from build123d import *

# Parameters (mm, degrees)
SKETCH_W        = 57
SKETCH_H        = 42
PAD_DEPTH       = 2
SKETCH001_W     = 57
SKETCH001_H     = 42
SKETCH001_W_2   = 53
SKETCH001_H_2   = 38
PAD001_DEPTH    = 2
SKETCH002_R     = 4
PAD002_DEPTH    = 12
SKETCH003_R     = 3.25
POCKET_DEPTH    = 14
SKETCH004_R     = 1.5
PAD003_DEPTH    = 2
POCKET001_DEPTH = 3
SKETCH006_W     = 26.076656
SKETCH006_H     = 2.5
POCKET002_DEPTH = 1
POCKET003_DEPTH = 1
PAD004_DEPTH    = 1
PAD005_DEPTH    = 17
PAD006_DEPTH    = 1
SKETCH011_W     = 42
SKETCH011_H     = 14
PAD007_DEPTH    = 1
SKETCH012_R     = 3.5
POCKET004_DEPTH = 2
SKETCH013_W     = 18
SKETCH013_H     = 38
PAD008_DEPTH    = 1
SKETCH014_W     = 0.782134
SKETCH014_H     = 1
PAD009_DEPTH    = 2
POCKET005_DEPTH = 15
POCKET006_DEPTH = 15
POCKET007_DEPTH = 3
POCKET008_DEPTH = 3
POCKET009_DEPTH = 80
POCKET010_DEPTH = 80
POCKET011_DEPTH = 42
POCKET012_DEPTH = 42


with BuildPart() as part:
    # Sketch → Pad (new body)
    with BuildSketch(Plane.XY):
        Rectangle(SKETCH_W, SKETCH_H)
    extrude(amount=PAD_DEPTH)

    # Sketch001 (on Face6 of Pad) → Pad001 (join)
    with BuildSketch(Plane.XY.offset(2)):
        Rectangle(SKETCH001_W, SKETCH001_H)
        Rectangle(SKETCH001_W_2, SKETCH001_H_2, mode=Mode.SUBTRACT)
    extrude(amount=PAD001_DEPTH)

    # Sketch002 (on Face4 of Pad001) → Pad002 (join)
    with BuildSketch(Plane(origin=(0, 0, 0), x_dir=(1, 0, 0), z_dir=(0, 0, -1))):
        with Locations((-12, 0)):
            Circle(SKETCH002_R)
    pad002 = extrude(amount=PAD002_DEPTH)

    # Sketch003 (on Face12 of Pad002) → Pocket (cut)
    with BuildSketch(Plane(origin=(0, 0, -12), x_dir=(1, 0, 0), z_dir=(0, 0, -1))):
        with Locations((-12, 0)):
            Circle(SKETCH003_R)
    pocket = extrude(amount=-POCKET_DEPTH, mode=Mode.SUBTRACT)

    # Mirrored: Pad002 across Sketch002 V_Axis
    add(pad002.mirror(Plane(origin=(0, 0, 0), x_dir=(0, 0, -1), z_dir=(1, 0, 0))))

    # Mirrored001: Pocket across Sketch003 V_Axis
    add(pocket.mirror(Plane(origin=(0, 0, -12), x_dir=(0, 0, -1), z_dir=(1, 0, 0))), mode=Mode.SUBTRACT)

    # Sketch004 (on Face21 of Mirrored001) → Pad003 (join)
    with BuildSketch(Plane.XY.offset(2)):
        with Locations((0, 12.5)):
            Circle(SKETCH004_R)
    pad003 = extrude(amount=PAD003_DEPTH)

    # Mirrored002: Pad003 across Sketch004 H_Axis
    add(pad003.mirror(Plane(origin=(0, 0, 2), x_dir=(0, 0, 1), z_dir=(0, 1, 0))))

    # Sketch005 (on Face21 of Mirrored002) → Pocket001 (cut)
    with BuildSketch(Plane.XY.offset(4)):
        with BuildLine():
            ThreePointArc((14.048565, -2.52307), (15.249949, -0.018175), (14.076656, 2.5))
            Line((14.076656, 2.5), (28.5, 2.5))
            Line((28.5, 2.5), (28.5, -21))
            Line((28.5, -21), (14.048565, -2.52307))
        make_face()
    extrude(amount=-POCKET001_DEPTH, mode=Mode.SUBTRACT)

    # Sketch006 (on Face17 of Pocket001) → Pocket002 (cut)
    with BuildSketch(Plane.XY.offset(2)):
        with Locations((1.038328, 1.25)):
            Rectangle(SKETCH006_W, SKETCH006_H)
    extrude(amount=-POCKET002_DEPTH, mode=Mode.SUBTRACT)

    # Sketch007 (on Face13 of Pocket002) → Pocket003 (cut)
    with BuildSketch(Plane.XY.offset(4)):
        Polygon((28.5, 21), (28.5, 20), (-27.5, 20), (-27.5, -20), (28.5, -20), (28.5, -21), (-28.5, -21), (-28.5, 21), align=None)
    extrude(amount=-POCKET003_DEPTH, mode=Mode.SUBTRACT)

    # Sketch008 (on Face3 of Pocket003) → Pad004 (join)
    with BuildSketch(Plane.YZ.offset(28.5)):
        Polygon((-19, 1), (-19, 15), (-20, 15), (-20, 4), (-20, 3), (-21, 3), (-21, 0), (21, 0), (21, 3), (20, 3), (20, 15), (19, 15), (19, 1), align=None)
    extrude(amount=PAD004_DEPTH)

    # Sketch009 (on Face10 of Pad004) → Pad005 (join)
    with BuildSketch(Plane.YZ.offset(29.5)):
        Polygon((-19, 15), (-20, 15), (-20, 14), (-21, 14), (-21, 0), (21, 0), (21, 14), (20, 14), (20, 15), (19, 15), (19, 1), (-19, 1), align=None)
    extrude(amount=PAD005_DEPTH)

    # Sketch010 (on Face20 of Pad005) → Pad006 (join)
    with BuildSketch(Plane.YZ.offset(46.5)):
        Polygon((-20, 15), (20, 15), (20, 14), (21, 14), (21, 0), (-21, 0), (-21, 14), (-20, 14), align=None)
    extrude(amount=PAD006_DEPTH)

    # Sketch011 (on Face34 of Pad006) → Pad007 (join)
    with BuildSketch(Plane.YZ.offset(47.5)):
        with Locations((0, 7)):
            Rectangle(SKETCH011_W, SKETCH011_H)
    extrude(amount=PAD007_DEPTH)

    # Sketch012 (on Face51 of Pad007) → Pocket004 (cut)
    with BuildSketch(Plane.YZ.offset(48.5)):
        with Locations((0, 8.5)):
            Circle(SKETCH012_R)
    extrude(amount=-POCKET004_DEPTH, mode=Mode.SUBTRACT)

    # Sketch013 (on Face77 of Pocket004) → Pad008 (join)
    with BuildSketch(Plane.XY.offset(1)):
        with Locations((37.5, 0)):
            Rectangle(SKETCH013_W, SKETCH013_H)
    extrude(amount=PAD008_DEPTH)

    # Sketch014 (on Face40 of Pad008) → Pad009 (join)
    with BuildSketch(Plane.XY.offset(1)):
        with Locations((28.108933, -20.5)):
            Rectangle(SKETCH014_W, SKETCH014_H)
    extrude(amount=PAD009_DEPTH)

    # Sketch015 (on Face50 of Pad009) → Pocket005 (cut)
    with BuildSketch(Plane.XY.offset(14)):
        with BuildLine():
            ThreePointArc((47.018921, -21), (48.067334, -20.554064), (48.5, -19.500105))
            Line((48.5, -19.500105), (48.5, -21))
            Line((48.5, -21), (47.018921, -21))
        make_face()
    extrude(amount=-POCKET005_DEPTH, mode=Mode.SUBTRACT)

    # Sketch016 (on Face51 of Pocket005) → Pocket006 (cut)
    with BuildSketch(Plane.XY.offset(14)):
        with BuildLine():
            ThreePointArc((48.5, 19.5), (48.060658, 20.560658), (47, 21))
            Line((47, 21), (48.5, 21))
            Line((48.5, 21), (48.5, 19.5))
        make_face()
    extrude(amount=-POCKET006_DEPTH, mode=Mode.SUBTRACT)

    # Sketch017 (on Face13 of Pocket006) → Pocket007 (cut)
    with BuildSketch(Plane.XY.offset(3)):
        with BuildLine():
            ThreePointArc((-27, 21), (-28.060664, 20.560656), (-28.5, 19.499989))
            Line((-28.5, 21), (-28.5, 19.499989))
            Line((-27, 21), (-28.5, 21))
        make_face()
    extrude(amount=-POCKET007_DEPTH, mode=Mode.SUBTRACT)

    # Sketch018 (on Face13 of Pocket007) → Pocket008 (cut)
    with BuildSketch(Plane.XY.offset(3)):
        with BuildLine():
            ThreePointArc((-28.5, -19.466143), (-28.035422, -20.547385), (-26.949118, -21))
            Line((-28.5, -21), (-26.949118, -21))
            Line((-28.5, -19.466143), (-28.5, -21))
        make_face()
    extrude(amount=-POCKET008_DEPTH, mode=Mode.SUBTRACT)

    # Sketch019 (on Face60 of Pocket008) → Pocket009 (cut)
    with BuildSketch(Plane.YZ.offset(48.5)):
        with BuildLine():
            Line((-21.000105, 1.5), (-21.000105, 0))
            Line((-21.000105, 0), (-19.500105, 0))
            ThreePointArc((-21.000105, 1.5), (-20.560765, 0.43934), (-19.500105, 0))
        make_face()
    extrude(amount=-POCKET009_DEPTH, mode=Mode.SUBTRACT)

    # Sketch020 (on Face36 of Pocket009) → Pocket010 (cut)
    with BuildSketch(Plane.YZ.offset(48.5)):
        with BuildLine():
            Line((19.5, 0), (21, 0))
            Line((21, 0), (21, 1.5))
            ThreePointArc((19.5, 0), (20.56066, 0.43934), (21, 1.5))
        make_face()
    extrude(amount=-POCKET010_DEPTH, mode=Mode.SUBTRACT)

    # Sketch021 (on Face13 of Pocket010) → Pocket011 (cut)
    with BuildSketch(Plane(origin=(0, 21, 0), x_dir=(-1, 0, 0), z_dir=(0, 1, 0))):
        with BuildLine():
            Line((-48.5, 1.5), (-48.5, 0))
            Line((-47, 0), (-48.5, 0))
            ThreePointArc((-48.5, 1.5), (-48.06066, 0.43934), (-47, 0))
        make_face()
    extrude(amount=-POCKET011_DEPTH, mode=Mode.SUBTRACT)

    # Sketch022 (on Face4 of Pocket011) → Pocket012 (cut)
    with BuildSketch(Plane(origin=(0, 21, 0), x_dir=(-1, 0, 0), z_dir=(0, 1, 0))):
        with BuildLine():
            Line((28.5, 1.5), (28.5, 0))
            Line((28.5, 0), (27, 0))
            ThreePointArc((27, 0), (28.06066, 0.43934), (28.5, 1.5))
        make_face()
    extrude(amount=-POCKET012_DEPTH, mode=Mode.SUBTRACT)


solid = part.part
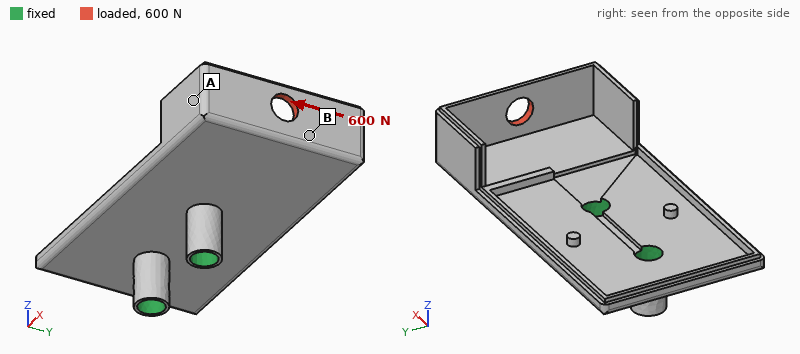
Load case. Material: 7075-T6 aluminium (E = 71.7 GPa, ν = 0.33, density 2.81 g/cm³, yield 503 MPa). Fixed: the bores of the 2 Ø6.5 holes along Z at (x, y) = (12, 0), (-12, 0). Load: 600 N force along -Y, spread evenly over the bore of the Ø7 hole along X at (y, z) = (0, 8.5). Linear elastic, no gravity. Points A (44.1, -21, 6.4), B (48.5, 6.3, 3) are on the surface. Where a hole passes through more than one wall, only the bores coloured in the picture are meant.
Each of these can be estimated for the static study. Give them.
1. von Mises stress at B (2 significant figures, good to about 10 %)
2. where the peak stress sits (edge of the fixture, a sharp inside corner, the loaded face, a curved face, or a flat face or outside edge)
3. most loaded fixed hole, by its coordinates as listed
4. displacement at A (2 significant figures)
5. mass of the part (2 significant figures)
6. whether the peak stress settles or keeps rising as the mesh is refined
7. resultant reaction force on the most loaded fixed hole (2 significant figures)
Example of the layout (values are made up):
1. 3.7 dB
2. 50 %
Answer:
1. 80 MPa
2. edge of the fixture
3. (12, 0)
4. 0.75 mm
5. 25 g
6. keeps rising
7. 1.3 kN
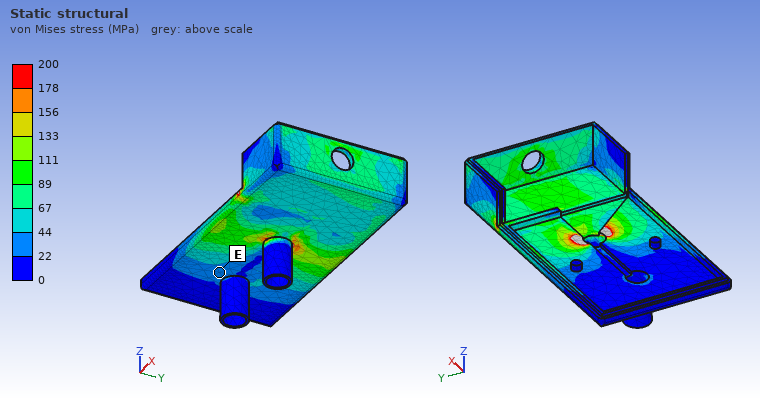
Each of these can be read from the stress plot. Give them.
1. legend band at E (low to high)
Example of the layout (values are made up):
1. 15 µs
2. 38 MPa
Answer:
1. 22 to 44 MPa
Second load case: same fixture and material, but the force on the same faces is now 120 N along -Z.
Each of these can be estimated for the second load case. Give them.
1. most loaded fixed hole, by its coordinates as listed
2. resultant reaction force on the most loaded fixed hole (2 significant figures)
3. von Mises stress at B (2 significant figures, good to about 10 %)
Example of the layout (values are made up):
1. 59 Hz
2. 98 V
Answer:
1. (12, 0)
2. 300 N
3. 18 MPa
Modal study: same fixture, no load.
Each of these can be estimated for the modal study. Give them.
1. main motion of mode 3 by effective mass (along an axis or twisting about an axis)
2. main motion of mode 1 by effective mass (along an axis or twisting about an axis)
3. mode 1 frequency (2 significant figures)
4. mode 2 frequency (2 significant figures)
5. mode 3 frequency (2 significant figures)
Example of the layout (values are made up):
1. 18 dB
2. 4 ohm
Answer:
1. along Z
2. along Z
3. 760 Hz
4. 1200 Hz
5. 3700 Hz
